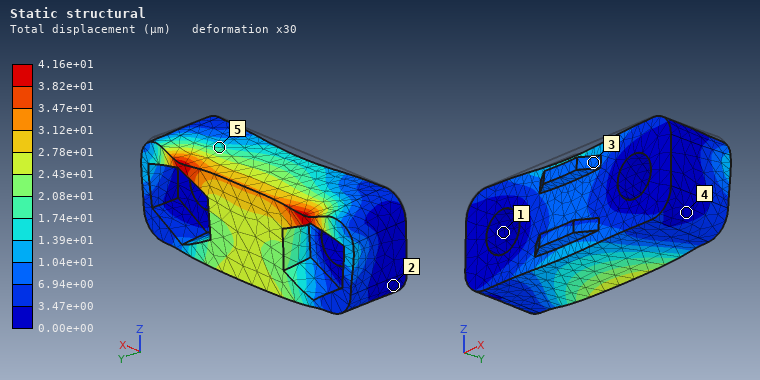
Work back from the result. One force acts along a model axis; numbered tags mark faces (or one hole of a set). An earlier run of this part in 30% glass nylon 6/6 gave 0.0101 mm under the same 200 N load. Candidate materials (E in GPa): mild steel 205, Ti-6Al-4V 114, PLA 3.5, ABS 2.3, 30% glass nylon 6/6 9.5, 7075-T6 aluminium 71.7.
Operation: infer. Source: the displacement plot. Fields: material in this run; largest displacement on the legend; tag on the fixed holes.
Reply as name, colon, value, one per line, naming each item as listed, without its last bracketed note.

material in this run: ABS
largest displacement on the legend: 4.16e+01 µm
tag on the fixed holes: 1
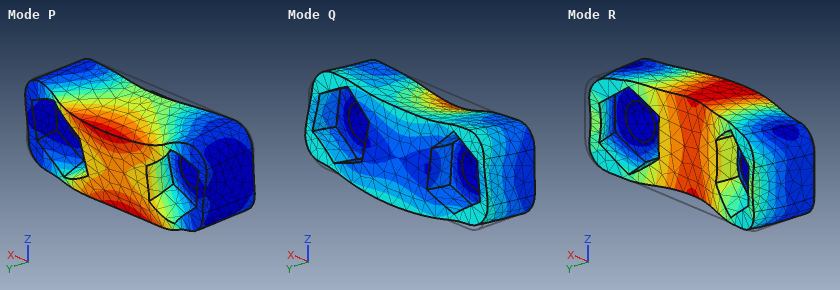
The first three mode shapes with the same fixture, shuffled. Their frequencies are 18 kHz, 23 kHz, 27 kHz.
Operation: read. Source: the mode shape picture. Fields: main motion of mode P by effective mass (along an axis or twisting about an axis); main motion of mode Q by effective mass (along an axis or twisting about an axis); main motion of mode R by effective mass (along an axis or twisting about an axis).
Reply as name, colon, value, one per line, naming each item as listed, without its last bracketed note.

main motion of mode P by effective mass: along Z
main motion of mode Q by effective mass: along Z
main motion of mode R by effective mass: along Y
